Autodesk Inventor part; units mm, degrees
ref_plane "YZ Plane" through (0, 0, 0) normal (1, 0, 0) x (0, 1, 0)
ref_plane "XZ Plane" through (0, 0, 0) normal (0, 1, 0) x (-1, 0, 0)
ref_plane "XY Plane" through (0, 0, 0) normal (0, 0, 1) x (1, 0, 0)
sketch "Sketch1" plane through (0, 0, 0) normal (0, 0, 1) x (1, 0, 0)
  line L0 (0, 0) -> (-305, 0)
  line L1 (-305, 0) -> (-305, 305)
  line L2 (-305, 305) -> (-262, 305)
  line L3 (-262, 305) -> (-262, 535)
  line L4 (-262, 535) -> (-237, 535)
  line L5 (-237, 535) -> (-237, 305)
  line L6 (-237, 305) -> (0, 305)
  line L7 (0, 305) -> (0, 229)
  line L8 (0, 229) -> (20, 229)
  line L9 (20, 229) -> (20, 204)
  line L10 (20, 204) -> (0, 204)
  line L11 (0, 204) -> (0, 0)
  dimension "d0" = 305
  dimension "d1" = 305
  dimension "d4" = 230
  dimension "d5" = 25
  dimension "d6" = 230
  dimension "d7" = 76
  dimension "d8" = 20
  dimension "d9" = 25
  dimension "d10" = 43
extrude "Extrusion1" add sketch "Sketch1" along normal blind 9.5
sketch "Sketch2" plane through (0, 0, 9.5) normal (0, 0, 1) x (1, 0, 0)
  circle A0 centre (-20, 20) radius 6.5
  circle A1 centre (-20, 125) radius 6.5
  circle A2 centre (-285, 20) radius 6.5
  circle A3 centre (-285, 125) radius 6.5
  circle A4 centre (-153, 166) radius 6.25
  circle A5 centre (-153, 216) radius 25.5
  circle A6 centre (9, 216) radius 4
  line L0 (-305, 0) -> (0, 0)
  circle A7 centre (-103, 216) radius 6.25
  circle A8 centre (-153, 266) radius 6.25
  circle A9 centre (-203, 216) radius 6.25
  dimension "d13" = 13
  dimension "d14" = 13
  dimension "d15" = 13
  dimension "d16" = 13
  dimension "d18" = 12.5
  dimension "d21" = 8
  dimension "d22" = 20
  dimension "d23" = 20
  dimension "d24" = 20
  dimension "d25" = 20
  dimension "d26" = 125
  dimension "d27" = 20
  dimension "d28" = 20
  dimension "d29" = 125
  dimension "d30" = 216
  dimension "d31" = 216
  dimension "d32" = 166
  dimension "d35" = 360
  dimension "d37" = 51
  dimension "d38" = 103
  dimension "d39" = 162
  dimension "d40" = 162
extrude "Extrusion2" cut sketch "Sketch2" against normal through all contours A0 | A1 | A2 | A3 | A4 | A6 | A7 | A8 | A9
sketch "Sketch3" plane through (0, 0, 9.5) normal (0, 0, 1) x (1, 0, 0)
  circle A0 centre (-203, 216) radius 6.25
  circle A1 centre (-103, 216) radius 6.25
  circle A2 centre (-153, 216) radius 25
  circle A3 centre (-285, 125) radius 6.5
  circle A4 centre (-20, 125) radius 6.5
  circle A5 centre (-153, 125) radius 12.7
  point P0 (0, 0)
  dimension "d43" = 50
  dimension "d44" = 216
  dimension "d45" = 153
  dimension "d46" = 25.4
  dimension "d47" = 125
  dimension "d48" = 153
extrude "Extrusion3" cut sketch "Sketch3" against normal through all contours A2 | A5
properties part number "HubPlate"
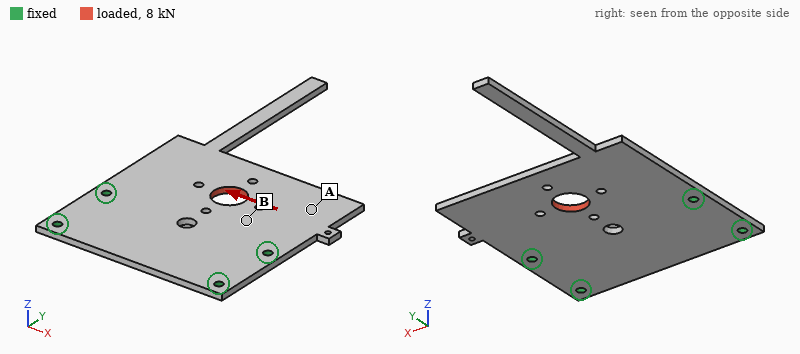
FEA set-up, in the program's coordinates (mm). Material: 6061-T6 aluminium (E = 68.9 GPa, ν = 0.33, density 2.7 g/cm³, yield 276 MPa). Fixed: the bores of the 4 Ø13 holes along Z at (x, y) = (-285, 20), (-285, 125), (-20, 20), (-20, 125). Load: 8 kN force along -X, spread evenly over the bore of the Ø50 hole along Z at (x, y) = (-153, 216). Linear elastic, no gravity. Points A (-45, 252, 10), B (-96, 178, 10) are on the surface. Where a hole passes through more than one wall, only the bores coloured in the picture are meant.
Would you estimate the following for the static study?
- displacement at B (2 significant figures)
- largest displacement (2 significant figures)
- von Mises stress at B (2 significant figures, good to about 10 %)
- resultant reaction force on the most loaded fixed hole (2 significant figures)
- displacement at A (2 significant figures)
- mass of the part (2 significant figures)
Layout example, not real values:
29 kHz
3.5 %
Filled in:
11 µm
39 µm
5.8 MPa
4.2 kN
19 µm
2.5 kg
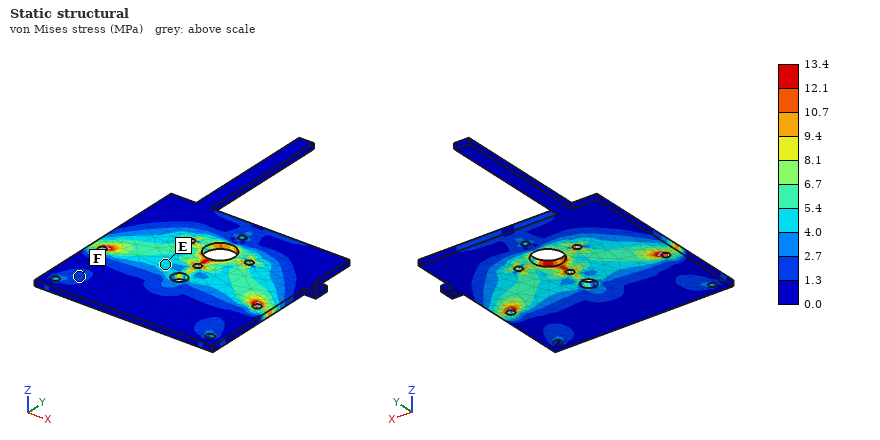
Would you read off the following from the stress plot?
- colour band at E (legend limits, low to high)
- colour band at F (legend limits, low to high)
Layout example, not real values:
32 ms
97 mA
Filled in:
4.0 to 5.4 MPa
1.3 to 2.7 MPa
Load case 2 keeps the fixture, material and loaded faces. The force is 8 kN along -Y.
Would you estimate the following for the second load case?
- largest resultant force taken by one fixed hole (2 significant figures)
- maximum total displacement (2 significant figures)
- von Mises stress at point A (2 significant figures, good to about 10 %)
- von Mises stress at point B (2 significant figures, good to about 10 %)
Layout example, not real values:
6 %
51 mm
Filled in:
2.9 kN
23 µm
1.3 MPa
3.9 MPa
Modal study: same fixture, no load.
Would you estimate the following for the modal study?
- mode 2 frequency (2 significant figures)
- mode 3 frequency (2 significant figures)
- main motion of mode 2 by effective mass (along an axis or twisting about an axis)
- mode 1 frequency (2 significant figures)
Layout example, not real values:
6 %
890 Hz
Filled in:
230 Hz
350 Hz
along Z
91 Hz
